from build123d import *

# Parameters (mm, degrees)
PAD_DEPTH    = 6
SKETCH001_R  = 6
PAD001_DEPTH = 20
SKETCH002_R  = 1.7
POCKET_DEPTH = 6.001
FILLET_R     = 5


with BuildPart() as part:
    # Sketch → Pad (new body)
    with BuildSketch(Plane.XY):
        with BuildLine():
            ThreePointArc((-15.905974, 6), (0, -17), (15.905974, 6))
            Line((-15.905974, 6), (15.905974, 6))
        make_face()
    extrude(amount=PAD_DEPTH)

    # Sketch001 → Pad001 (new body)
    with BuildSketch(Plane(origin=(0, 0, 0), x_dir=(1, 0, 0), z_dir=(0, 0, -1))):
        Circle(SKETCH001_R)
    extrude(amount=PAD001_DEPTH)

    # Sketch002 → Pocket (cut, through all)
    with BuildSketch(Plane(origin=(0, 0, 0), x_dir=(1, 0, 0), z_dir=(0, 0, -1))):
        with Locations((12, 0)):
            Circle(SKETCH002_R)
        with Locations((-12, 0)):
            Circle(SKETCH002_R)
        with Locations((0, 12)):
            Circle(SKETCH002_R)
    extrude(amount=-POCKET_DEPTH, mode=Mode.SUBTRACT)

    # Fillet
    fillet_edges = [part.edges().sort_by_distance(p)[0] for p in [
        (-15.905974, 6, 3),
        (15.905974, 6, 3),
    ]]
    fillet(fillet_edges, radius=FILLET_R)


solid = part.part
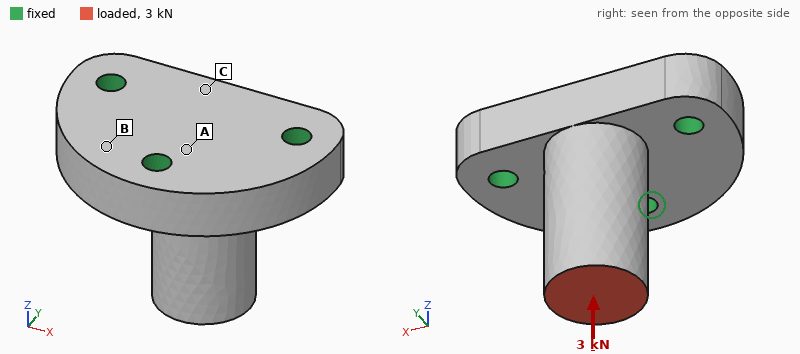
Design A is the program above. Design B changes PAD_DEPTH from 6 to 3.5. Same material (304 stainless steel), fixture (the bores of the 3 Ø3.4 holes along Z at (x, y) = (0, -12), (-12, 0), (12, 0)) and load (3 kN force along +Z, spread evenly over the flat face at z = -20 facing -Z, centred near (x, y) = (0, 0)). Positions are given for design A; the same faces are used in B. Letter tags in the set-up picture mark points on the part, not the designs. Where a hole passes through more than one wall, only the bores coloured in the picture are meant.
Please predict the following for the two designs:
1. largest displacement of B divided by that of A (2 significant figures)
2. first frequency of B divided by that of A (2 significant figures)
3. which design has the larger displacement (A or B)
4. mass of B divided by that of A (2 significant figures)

2.4
0.73
B
0.74
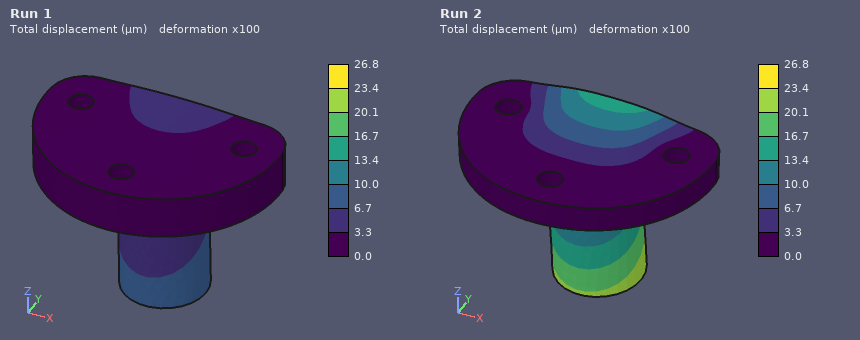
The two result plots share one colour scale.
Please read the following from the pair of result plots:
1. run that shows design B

Run 2
